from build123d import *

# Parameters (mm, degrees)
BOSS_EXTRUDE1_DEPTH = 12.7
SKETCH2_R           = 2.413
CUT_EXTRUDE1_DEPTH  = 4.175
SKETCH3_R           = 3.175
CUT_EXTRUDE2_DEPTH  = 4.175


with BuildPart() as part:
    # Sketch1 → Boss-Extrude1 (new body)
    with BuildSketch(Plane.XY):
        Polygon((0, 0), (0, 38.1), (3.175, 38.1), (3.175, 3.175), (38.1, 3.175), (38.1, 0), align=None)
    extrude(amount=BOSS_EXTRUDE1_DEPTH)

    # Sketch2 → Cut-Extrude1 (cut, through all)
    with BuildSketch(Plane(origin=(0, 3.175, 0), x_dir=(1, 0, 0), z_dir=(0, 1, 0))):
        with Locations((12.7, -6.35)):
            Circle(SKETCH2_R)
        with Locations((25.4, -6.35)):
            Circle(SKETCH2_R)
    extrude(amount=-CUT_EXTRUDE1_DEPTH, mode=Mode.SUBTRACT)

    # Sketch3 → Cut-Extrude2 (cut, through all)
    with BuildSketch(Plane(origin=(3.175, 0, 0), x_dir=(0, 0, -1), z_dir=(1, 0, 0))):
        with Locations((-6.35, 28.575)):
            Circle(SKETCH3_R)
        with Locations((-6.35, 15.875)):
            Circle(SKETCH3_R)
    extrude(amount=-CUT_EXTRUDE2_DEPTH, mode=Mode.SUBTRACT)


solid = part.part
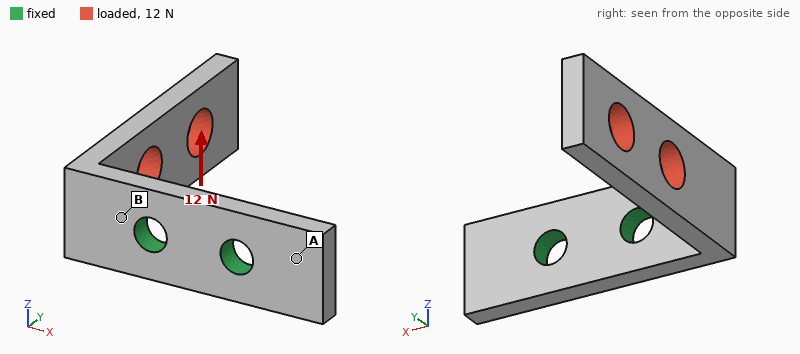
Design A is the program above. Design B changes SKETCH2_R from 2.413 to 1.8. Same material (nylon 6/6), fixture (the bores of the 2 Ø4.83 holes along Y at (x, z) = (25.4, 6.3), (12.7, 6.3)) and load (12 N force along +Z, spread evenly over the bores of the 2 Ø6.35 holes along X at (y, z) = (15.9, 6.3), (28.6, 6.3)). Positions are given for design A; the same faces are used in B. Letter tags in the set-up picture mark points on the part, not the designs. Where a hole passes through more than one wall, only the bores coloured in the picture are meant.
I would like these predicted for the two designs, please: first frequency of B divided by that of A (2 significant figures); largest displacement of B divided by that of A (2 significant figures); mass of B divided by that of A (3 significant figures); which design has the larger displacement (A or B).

0.98
1.1
1.02
B
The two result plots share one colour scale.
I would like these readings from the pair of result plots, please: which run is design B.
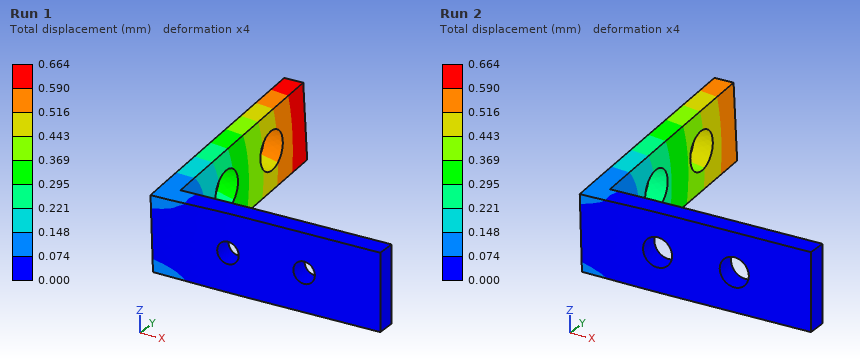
Run 1
